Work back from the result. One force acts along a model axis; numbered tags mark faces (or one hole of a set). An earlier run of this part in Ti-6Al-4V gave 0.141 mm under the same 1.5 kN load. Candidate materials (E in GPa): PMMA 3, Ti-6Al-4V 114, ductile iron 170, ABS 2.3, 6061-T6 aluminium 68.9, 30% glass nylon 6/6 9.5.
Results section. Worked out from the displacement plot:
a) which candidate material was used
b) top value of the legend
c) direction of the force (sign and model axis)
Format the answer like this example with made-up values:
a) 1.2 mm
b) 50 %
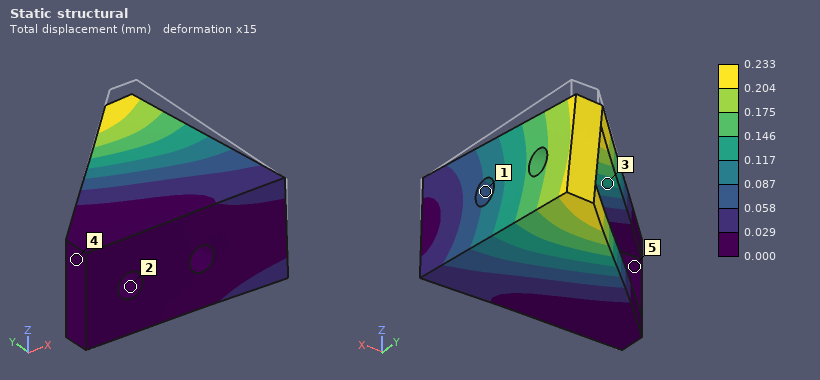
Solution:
a) 6061-T6 aluminium
b) 0.233 mm
c) -Z
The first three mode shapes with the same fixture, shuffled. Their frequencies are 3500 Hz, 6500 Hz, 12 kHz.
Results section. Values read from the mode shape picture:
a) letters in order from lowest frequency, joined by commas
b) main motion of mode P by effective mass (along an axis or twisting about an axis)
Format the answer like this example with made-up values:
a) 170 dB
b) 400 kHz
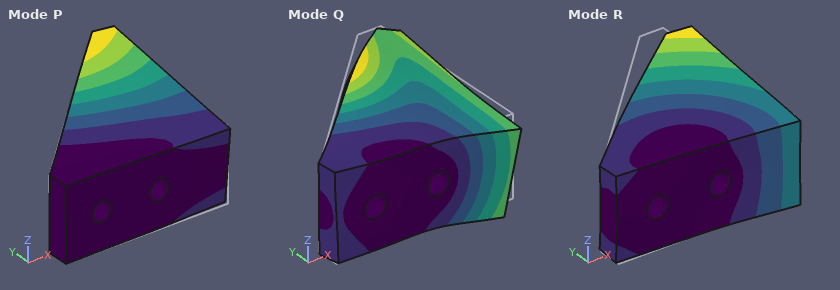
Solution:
a) P, R, Q
b) along Z
